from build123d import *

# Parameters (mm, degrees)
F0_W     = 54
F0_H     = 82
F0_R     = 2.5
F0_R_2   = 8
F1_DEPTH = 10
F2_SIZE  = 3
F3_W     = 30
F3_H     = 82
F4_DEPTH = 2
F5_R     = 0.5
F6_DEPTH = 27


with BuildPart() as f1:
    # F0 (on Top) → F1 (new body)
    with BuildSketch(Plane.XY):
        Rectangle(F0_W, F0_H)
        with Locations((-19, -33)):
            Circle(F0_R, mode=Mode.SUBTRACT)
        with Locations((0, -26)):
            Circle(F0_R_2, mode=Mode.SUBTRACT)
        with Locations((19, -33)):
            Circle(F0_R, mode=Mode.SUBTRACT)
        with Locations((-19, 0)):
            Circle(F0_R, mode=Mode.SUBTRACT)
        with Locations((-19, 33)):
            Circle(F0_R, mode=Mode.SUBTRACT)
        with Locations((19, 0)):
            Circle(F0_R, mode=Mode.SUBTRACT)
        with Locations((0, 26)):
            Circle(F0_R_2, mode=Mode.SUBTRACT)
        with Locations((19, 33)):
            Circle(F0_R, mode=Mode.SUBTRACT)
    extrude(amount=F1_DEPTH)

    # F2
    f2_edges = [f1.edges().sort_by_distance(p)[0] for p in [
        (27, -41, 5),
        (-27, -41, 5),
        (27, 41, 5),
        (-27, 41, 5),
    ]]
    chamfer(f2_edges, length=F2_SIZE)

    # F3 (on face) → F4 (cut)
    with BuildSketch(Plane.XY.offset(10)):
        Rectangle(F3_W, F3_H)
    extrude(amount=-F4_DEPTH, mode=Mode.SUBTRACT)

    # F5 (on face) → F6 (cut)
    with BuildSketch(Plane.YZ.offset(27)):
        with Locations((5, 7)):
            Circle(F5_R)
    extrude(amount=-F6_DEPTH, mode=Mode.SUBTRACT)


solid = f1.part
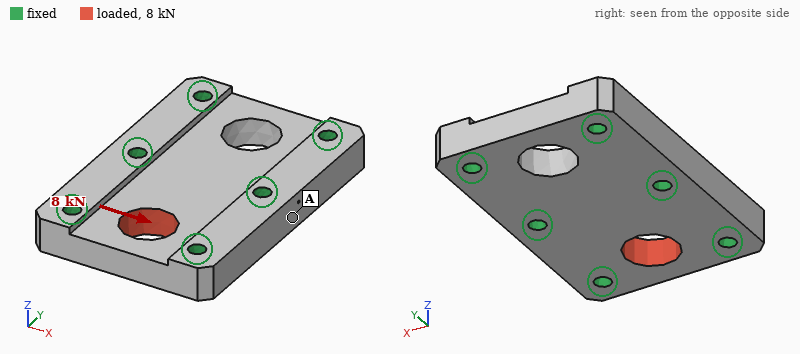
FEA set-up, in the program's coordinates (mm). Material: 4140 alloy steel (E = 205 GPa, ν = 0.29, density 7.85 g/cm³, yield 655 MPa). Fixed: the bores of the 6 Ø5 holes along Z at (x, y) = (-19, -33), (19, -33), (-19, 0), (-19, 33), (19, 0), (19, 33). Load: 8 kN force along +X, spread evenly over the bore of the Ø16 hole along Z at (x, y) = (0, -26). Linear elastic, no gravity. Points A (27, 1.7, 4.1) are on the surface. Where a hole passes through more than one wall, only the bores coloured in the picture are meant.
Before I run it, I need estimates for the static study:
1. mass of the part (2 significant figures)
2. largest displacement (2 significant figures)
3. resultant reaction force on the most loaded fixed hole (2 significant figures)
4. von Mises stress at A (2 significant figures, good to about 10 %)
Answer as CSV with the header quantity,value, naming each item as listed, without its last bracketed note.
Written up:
quantity,value
mass of the part,270 g
largest displacement,2.0 µm
resultant reaction force on the most loaded fixed hole,2.9 kN
von Mises stress at A,6.4 MPa
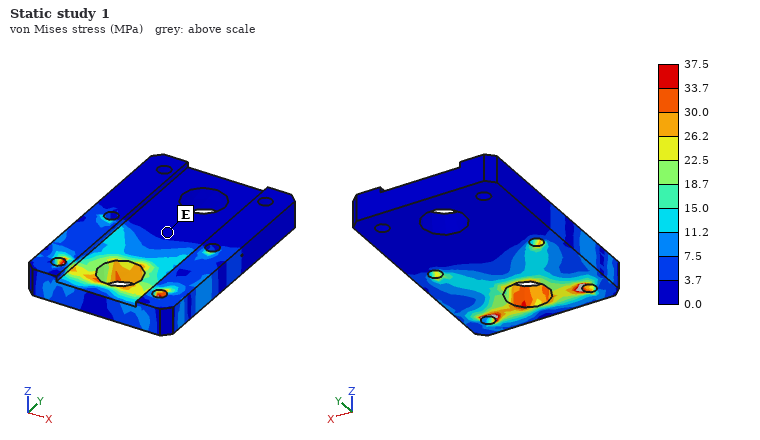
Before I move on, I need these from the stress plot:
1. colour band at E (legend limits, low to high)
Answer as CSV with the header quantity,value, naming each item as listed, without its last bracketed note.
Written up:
quantity,value
colour band at E,0.0 to 3.7 MPa
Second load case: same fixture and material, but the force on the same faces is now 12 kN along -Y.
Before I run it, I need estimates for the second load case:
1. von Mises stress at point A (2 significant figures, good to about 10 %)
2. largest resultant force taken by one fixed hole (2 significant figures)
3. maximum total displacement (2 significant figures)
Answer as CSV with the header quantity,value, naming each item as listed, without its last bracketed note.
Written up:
quantity,value
von Mises stress at point A,7.4 MPa
largest resultant force taken by one fixed hole,3.4 kN
maximum total displacement,7.5 µm
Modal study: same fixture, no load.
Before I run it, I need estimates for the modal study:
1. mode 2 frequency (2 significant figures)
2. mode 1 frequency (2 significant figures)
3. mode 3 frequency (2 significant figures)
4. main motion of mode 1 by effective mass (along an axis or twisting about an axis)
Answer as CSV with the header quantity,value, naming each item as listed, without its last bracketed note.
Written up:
quantity,value
mode 2 frequency,25 kHz
mode 1 frequency,22 kHz
mode 3 frequency,30 kHz
main motion of mode 1 by effective mass,along Z
